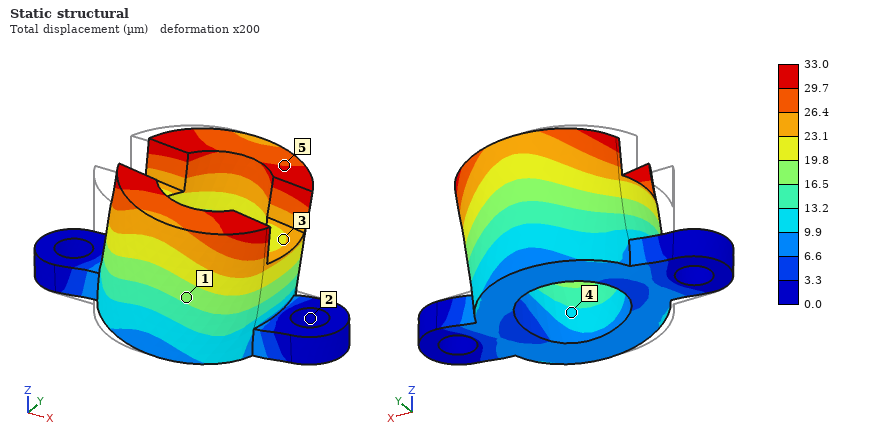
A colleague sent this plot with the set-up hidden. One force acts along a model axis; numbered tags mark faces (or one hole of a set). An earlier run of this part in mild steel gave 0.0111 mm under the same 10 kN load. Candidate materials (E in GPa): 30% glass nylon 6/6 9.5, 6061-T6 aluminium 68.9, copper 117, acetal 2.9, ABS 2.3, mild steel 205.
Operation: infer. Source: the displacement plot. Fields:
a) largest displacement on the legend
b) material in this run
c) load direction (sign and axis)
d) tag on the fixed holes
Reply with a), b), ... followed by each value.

a) 33.0 µm
b) 6061-T6 aluminium
c) +X
d) 2
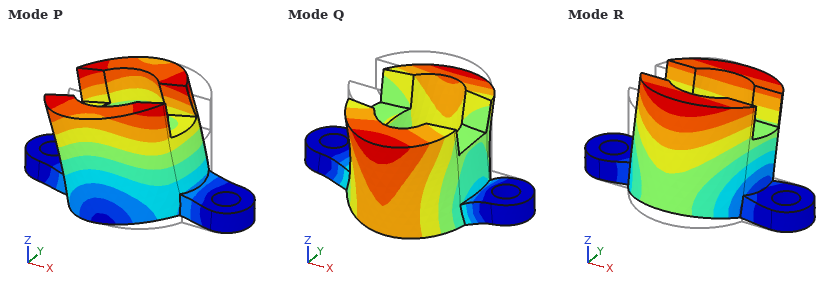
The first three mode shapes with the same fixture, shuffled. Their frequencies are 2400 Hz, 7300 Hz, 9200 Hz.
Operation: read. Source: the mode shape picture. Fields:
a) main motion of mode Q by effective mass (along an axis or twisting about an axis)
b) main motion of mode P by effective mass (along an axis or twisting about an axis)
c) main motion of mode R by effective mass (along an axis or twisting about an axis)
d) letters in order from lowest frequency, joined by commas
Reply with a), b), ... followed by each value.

a) along Z
b) along X
c) along Y
d) R, Q, P
